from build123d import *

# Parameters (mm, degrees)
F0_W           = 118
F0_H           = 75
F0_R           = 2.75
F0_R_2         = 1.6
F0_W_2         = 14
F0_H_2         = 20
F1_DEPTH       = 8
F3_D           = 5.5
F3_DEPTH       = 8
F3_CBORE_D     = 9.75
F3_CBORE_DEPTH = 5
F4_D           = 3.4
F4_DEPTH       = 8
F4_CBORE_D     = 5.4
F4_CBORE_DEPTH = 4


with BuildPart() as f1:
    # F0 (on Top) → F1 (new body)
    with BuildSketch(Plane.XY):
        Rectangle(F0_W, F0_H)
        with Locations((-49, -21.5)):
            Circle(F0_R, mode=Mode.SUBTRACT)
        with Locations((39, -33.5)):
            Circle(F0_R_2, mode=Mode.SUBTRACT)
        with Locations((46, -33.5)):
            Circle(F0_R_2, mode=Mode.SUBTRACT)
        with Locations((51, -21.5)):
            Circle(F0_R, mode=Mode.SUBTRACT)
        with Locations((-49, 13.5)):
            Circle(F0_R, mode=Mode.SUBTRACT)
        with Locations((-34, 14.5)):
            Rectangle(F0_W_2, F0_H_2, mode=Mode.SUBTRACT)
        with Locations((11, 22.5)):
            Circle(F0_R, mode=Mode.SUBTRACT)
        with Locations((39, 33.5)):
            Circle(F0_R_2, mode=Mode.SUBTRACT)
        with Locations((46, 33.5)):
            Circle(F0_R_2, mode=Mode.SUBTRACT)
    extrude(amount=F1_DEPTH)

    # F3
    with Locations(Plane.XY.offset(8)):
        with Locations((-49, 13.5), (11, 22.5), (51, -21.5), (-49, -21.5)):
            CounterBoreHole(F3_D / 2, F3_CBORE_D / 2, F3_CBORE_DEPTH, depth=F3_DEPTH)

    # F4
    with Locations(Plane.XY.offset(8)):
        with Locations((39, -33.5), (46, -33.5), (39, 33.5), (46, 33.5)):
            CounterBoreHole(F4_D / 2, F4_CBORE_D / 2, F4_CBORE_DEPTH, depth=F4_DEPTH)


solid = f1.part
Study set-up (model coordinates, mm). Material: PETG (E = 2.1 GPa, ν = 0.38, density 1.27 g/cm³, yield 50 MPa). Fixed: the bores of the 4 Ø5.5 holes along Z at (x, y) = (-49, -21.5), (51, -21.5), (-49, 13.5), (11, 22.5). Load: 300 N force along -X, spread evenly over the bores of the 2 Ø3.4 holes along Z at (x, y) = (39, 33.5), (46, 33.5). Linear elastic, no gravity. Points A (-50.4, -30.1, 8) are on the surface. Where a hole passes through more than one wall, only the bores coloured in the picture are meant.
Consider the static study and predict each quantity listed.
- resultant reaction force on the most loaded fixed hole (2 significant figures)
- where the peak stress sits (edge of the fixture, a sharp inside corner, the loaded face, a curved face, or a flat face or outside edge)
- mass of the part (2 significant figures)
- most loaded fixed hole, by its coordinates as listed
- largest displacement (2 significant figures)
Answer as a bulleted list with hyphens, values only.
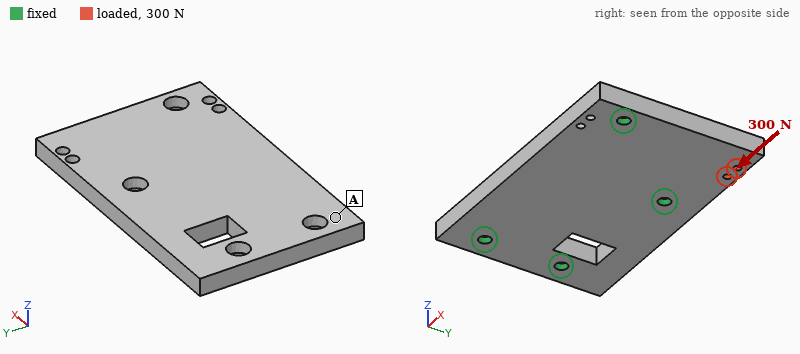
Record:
- 240 N
- the loaded face
- 84 g
- (11, 22.5)
- 0.14 mm
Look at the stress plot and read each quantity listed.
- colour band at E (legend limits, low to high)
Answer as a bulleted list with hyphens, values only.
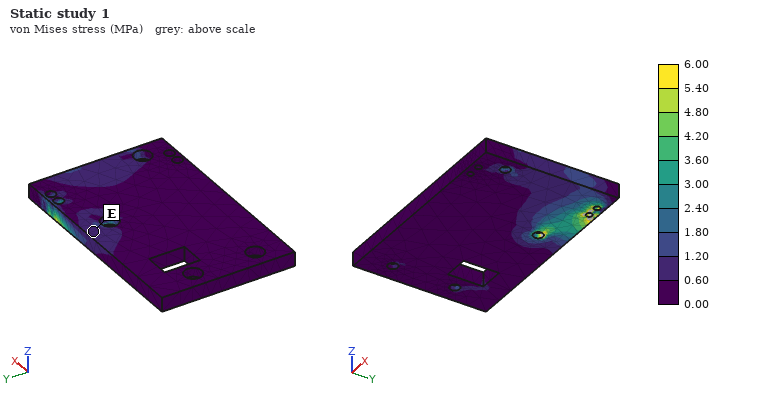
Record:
- 0.60 to 1.20 MPa
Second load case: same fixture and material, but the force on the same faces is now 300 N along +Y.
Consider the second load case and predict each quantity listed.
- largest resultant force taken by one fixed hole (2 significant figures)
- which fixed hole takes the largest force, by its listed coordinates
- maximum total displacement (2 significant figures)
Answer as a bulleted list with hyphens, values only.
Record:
- 180 N
- (51, -21.5)
- 99 µm
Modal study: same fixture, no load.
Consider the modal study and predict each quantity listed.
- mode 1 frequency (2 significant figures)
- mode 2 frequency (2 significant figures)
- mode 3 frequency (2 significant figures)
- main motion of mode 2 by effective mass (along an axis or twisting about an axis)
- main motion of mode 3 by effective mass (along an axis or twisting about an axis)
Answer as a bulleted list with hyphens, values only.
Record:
- 770 Hz
- 1000 Hz
- 1500 Hz
- along Z
- along Z
